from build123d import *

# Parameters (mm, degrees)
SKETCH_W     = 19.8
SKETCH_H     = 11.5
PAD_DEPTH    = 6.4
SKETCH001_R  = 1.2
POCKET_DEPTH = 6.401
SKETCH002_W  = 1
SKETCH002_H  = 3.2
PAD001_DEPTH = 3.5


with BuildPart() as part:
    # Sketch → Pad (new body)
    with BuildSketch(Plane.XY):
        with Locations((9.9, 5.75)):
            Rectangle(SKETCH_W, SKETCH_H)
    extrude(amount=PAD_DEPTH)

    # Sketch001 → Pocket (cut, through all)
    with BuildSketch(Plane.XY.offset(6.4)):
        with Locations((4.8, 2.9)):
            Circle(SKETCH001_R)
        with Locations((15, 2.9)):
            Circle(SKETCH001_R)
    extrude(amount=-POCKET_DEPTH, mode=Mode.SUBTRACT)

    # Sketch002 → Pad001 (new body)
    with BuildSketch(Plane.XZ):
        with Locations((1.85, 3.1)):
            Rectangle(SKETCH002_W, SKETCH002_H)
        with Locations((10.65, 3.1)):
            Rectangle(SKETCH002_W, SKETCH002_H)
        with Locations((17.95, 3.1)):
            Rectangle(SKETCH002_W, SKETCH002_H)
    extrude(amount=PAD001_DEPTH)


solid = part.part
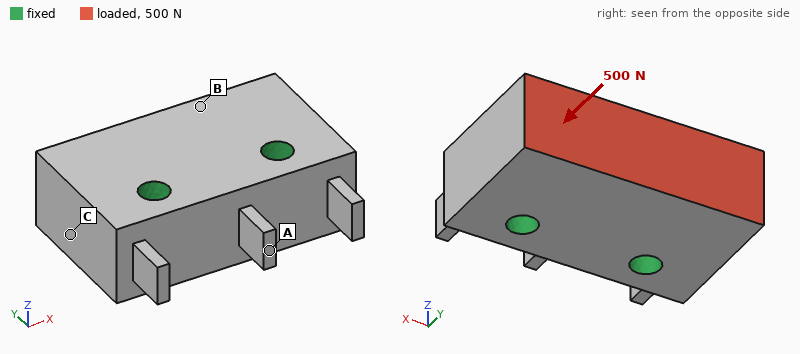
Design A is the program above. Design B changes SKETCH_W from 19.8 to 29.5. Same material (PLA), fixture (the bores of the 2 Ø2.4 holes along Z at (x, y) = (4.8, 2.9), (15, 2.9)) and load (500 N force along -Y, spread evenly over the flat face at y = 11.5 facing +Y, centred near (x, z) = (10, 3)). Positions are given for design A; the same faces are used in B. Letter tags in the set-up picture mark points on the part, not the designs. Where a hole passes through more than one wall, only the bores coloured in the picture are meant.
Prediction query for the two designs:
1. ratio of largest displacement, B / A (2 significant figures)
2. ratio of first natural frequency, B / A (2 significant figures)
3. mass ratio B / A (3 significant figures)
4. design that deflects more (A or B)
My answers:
2.2
0.70
1.50
B
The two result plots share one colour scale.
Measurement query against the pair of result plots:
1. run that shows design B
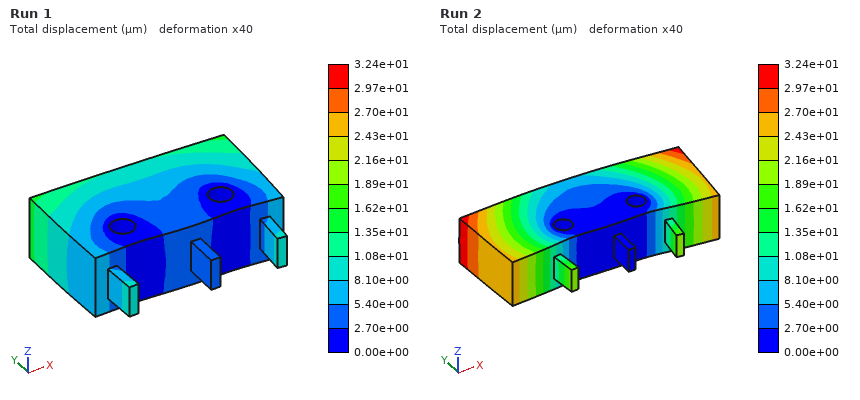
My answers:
Run 2
